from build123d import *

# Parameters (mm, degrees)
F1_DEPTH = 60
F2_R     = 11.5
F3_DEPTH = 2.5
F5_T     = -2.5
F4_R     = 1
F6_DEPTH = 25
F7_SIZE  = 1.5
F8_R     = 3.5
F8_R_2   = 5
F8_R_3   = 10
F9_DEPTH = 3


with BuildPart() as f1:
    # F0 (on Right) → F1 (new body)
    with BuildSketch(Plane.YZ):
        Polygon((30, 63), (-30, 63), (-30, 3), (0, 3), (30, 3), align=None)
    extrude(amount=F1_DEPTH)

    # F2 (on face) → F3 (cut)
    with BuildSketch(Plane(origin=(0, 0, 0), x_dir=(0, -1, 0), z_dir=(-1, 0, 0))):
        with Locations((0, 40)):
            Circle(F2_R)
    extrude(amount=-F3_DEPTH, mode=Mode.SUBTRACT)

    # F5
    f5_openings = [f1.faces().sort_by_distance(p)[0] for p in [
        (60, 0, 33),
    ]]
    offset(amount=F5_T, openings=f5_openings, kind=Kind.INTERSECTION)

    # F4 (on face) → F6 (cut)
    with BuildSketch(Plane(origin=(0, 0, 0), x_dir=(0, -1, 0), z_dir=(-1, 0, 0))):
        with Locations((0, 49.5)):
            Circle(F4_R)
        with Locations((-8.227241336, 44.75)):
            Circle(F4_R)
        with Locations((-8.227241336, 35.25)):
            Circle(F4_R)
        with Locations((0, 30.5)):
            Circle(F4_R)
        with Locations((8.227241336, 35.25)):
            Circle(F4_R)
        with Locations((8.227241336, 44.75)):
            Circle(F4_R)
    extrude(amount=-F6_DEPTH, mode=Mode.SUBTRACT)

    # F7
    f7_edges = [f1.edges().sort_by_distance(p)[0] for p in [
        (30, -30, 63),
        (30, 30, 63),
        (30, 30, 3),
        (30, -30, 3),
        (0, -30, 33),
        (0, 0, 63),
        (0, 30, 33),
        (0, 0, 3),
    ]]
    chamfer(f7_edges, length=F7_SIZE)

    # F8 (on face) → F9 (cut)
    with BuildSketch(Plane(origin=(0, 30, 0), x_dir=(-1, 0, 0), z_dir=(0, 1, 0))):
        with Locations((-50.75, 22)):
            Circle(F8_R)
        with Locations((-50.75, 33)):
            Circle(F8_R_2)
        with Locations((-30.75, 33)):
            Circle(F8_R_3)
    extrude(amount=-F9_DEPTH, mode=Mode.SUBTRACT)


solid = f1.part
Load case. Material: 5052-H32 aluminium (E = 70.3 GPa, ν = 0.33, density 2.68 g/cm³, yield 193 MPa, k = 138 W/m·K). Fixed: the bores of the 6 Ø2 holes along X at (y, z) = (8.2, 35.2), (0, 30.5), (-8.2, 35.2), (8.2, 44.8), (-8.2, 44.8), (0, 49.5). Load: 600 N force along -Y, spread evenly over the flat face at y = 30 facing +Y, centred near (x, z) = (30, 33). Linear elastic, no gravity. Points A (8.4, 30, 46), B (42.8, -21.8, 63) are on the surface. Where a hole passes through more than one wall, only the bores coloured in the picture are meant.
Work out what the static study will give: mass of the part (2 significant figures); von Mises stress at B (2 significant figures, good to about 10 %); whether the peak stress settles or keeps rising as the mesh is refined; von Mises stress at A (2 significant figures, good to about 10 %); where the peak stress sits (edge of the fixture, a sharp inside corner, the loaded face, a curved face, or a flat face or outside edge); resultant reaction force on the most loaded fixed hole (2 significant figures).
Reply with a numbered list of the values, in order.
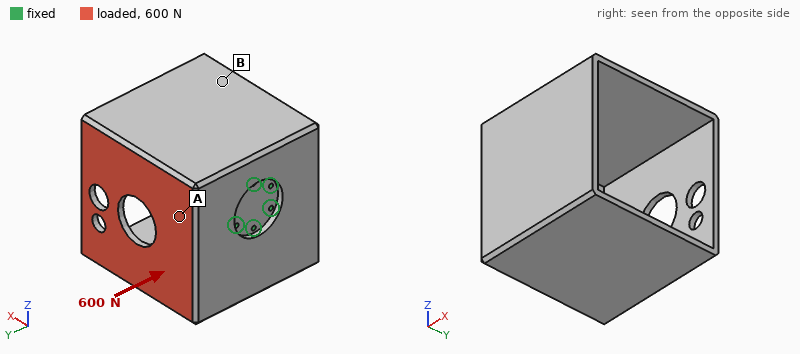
1. 110 g
2. 9.9 MPa
3. keeps rising
4. 23 MPa
5. edge of the fixture
6. 560 N
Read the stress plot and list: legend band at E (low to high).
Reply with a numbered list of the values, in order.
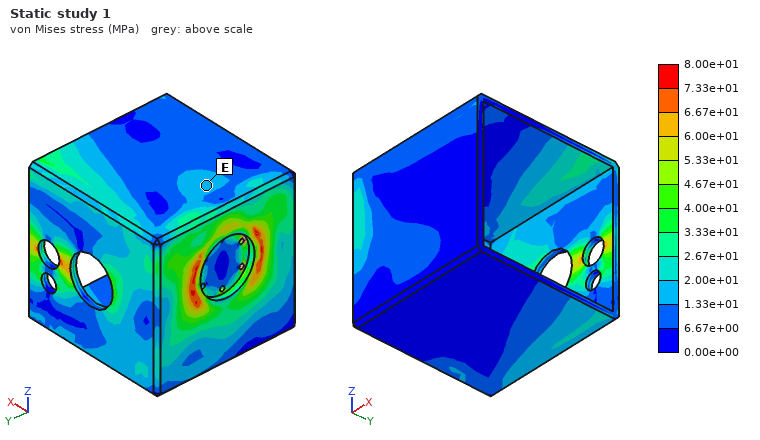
1. 1.33e+01 to 2.00e+01 MPa
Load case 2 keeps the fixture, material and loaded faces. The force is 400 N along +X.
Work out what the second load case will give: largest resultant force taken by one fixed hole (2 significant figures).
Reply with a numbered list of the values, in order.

1. 490 N
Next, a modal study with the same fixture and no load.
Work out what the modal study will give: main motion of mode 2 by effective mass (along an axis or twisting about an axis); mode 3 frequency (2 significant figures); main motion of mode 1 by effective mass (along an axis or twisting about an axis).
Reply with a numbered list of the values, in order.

1. along Y
2. 1300 Hz
3. along Z
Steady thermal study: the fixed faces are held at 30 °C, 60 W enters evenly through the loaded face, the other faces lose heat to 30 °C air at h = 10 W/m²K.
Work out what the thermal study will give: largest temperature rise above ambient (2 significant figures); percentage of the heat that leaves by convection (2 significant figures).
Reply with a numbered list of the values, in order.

1. 80 K
2. 18 %
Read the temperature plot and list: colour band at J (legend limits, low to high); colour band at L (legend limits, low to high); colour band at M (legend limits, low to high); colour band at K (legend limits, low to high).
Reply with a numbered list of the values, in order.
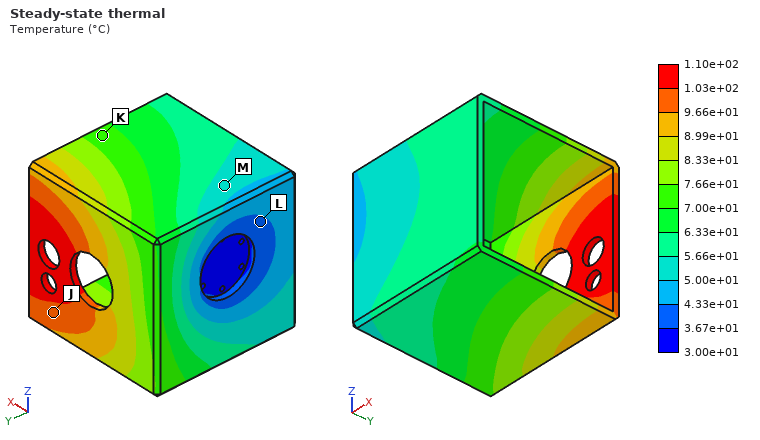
1. 9.66e+01 to 1.03e+02 °C
2. 3.67e+01 to 4.33e+01 °C
3. 5.00e+01 to 5.66e+01 °C
4. 7.00e+01 to 7.66e+01 °C
